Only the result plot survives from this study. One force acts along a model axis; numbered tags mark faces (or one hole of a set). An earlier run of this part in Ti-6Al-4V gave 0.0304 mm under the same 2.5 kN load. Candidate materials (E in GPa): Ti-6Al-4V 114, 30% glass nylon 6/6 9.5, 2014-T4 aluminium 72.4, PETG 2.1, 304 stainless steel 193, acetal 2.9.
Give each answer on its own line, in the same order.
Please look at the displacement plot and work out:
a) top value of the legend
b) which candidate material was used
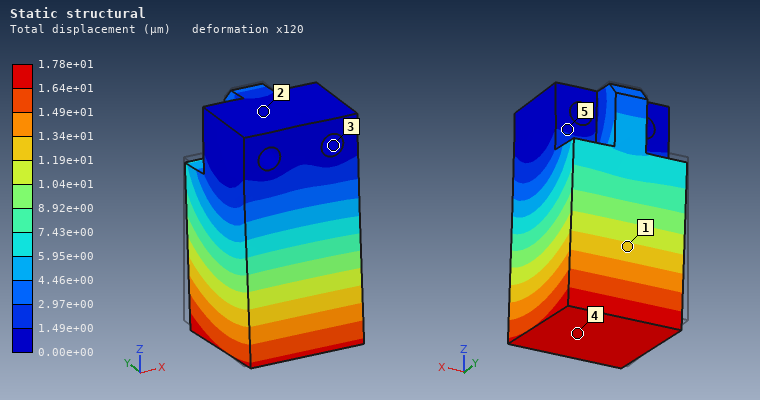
1.78e+01 µm
304 stainless steel
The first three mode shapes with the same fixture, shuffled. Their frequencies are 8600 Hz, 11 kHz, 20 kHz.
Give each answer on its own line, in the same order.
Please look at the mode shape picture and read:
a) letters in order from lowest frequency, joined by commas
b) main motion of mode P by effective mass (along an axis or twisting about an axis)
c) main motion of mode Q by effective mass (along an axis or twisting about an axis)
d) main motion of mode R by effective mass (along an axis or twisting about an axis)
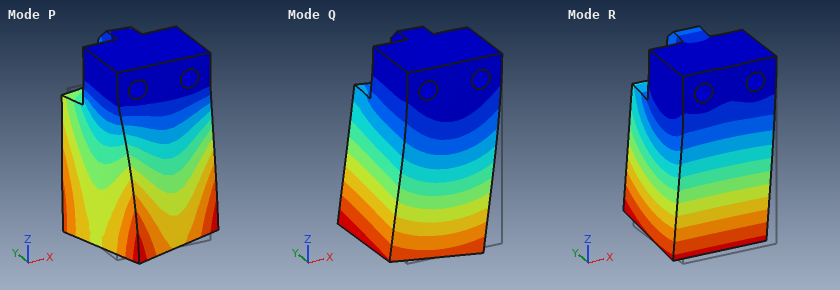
R, Q, P
twisting about Z
along X
along Y
